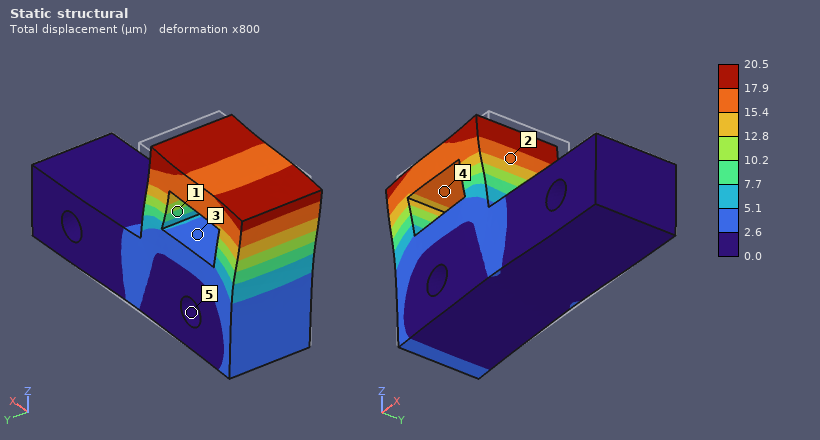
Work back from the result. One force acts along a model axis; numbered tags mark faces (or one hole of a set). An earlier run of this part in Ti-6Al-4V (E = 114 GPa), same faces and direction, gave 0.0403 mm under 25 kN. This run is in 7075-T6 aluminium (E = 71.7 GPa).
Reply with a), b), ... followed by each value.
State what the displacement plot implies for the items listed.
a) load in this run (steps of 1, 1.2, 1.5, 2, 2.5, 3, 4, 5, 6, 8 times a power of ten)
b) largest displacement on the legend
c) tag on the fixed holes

a) 8 kN
b) 20.5 µm
c) 5
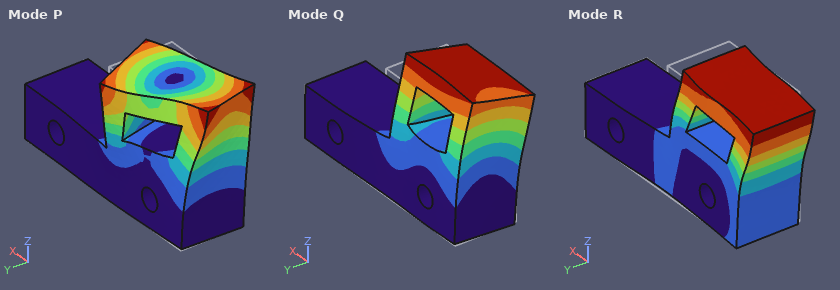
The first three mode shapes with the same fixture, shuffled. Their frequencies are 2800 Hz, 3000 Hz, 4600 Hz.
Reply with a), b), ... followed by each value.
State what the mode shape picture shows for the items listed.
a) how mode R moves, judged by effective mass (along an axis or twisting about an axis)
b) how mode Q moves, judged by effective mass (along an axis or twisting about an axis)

a) along X
b) along Y
